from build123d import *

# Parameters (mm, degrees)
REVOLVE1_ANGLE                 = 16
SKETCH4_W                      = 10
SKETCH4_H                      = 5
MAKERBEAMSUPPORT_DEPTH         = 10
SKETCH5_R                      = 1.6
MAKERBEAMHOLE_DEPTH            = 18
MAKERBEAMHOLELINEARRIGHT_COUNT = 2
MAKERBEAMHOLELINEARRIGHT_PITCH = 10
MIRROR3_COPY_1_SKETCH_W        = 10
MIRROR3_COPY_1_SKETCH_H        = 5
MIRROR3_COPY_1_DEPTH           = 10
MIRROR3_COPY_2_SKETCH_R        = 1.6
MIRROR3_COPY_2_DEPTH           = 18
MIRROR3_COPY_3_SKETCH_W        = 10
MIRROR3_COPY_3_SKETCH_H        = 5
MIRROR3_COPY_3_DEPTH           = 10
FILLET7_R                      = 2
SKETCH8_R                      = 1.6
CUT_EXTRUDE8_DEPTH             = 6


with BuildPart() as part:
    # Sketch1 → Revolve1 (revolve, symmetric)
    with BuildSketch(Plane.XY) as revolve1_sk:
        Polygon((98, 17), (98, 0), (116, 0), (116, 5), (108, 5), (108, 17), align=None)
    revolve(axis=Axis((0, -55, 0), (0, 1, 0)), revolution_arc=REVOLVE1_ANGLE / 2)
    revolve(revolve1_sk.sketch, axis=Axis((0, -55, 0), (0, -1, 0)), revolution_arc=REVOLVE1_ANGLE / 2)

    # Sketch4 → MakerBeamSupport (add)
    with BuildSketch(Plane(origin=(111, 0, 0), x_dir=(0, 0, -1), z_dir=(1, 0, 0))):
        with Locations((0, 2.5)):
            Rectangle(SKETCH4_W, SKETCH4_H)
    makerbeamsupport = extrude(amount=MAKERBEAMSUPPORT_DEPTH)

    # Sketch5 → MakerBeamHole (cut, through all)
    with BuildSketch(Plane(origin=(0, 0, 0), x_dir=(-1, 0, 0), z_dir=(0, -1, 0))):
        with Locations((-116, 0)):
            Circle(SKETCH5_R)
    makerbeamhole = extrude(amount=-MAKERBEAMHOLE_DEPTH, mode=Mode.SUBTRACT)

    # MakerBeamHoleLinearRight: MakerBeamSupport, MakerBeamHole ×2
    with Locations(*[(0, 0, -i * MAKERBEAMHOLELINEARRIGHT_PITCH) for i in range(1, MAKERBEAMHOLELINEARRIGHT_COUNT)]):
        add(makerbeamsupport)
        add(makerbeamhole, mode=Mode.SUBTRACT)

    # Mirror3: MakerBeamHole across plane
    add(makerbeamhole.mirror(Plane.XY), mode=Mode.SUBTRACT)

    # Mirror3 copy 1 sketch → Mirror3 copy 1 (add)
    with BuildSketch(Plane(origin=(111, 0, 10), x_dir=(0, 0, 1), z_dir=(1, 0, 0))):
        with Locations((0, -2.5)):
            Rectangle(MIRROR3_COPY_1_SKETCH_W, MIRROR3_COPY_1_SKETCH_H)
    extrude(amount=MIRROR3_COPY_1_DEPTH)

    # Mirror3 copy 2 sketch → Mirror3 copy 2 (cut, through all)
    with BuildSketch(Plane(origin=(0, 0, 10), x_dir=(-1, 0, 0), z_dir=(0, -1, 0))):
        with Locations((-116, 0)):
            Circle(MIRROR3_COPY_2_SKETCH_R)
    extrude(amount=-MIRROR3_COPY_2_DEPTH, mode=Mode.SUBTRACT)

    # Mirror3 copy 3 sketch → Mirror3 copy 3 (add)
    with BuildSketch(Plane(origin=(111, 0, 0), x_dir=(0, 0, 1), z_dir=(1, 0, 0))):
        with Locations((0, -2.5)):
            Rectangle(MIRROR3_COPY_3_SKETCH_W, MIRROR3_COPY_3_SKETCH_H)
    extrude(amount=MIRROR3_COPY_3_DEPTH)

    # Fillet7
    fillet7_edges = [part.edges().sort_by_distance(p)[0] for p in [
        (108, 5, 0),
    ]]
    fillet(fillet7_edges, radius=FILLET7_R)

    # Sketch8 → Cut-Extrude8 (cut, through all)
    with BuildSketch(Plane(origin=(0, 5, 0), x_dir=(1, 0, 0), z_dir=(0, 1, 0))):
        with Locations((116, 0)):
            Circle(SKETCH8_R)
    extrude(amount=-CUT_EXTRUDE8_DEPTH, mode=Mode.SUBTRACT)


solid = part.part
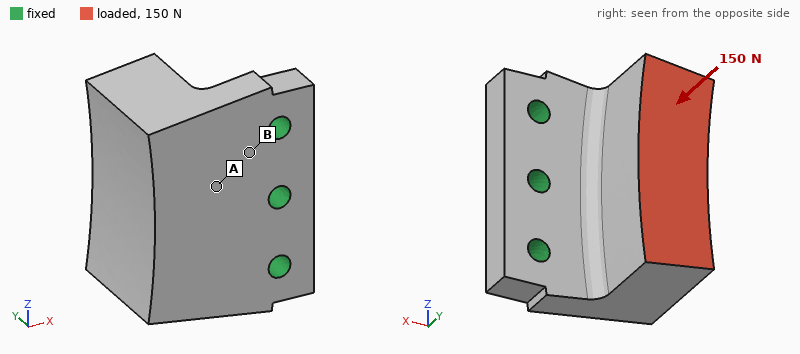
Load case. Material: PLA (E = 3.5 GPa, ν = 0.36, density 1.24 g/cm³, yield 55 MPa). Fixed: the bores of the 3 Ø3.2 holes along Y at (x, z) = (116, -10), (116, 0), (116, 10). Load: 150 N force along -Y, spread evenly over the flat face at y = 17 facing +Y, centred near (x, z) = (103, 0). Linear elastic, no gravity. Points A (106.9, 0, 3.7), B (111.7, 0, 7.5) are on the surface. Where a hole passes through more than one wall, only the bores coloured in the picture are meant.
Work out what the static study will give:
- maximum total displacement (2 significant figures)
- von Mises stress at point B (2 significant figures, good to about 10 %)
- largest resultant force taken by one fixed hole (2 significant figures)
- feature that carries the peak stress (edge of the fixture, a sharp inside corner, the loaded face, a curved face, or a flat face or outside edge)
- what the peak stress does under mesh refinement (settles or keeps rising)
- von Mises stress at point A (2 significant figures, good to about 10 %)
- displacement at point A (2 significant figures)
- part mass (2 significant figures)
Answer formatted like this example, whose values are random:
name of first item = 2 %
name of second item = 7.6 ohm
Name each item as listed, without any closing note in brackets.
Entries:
maximum total displacement = 0.21 mm
von Mises stress at point B = 9.1 MPa
largest resultant force taken by one fixed hole = 53 N
feature that carries the peak stress = edge of the fixture
what the peak stress does under mesh refinement = keeps rising
von Mises stress at point A = 3.5 MPa
displacement at point A = 0.062 mm
part mass = 8.5 g
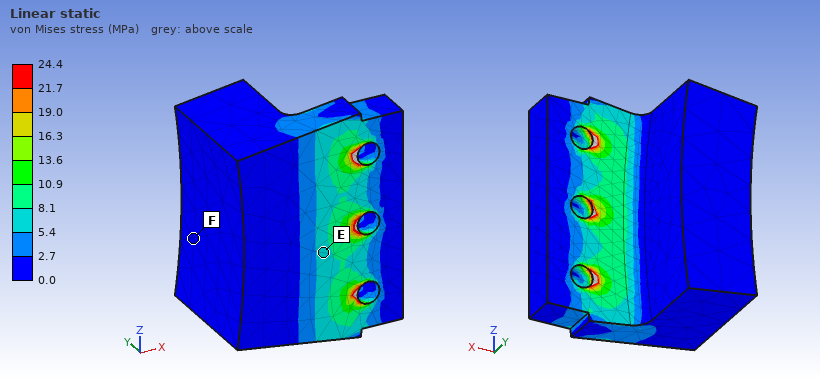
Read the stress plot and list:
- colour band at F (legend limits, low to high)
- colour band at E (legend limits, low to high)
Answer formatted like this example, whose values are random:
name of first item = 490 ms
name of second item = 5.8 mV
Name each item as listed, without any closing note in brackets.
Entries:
colour band at F = 0.0 to 2.7 MPa
colour band at E = 5.4 to 8.1 MPa
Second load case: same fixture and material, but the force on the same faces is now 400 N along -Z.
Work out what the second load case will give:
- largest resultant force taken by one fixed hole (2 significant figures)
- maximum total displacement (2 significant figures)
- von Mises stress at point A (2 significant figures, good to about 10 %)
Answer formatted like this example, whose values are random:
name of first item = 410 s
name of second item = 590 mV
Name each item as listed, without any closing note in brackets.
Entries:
largest resultant force taken by one fixed hole = 360 N
maximum total displacement = 0.24 mm
von Mises stress at point A = 4.9 MPa
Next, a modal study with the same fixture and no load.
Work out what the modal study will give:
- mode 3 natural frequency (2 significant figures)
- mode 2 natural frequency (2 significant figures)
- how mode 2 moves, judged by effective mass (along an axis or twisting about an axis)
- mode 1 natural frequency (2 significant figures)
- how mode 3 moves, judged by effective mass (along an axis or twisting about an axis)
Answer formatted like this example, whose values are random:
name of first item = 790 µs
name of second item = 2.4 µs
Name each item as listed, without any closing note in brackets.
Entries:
mode 3 natural frequency = 6800 Hz
mode 2 natural frequency = 4100 Hz
how mode 2 moves, judged by effective mass = along Z
mode 1 natural frequency = 1900 Hz
how mode 3 moves, judged by effective mass = along Z
